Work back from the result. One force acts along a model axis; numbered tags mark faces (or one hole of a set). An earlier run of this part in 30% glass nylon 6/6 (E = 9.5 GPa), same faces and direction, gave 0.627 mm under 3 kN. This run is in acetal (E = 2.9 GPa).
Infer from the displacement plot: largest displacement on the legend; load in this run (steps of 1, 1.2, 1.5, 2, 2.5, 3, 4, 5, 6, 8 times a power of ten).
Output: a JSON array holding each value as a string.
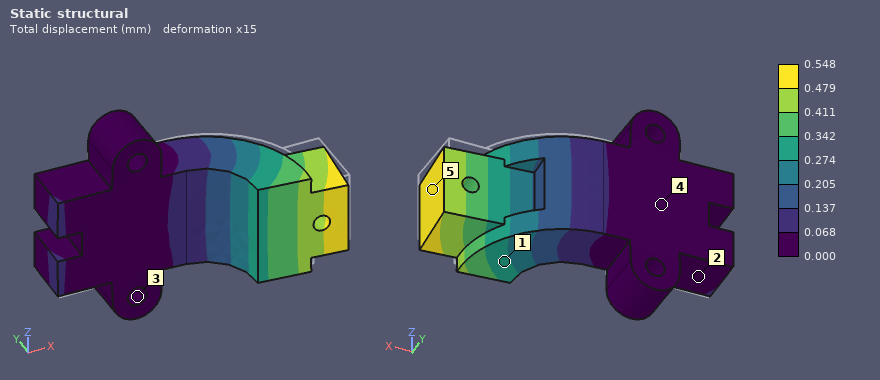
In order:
["0.548 mm", "800 N"]
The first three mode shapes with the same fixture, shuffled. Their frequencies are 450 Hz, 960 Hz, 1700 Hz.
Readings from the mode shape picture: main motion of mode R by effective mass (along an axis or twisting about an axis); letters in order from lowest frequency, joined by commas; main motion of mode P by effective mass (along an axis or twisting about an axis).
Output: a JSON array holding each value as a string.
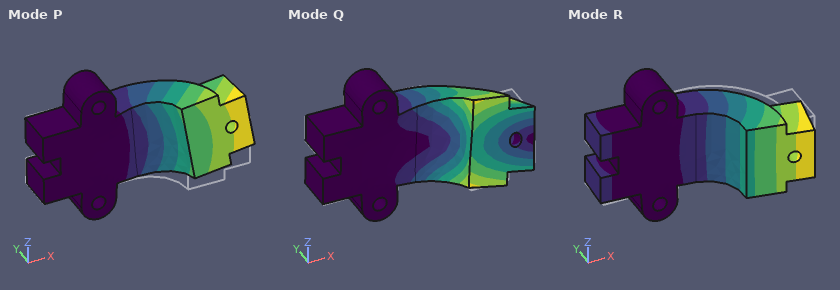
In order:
["along Y", "R, P, Q", "along Z"]
